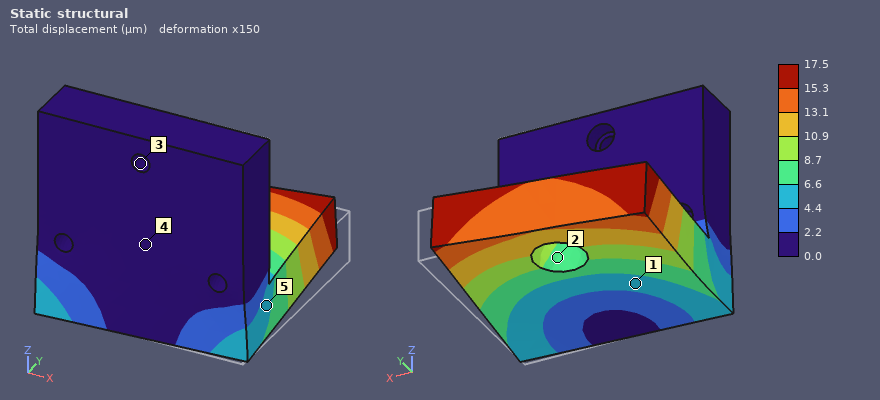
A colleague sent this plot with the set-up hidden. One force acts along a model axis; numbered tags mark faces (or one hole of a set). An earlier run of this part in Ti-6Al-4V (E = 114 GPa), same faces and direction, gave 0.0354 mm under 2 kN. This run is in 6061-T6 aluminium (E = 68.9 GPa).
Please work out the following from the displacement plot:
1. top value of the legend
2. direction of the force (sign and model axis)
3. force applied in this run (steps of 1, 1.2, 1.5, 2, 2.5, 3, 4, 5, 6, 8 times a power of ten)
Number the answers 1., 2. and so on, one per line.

1. 17.5 µm
2. -X
3. 600 N
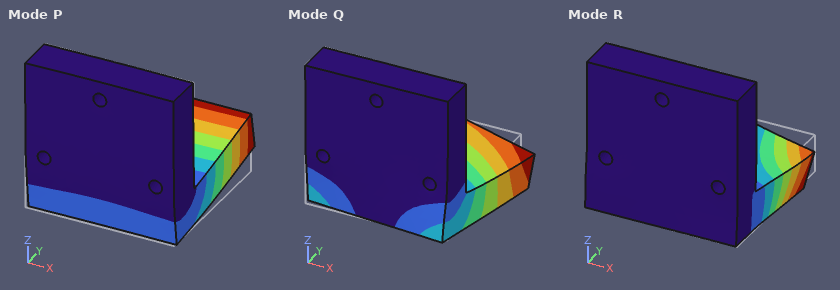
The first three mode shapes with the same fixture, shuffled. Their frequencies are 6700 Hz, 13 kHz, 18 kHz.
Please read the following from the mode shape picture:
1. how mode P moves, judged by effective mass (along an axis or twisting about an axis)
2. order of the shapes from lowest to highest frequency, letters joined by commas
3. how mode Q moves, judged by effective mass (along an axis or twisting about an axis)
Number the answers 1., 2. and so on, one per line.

1. along Z
2. P, Q, R
3. along X
